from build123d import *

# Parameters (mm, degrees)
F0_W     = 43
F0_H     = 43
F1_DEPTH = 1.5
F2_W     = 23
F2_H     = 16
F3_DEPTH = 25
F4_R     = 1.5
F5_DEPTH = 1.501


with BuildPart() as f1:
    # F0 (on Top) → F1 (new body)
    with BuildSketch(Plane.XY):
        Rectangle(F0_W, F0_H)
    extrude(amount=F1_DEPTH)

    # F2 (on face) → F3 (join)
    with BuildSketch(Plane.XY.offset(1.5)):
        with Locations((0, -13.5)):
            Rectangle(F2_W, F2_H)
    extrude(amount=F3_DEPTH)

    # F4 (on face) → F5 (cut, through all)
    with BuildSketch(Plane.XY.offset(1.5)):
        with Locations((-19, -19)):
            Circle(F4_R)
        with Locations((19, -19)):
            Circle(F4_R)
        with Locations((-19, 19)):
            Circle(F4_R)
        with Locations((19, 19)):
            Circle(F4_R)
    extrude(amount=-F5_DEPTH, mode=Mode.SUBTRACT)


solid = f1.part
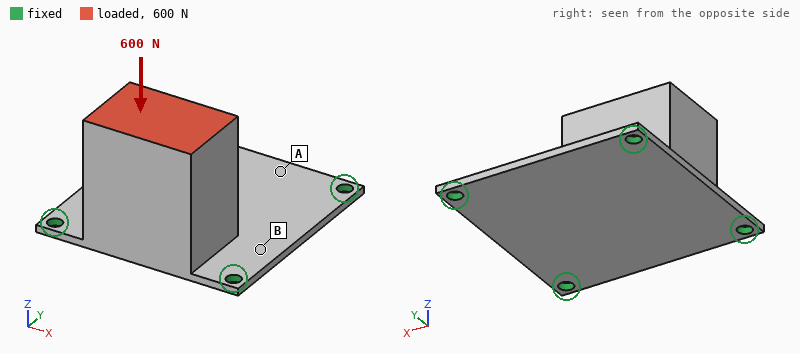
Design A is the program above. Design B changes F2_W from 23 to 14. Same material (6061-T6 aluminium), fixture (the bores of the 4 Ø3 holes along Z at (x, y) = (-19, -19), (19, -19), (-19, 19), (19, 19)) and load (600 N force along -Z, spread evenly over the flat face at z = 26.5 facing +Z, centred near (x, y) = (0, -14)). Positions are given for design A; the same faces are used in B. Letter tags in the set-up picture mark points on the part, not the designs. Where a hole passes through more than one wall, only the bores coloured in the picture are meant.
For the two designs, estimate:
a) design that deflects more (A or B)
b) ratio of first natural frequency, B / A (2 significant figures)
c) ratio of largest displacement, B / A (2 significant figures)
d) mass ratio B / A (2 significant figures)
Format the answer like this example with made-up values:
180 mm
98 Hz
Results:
B
1.1
1.2
0.70
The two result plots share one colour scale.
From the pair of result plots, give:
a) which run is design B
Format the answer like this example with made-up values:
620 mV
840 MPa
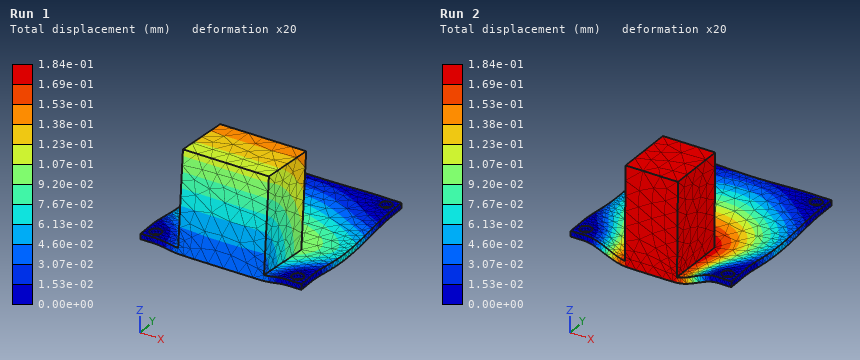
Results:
Run 2
